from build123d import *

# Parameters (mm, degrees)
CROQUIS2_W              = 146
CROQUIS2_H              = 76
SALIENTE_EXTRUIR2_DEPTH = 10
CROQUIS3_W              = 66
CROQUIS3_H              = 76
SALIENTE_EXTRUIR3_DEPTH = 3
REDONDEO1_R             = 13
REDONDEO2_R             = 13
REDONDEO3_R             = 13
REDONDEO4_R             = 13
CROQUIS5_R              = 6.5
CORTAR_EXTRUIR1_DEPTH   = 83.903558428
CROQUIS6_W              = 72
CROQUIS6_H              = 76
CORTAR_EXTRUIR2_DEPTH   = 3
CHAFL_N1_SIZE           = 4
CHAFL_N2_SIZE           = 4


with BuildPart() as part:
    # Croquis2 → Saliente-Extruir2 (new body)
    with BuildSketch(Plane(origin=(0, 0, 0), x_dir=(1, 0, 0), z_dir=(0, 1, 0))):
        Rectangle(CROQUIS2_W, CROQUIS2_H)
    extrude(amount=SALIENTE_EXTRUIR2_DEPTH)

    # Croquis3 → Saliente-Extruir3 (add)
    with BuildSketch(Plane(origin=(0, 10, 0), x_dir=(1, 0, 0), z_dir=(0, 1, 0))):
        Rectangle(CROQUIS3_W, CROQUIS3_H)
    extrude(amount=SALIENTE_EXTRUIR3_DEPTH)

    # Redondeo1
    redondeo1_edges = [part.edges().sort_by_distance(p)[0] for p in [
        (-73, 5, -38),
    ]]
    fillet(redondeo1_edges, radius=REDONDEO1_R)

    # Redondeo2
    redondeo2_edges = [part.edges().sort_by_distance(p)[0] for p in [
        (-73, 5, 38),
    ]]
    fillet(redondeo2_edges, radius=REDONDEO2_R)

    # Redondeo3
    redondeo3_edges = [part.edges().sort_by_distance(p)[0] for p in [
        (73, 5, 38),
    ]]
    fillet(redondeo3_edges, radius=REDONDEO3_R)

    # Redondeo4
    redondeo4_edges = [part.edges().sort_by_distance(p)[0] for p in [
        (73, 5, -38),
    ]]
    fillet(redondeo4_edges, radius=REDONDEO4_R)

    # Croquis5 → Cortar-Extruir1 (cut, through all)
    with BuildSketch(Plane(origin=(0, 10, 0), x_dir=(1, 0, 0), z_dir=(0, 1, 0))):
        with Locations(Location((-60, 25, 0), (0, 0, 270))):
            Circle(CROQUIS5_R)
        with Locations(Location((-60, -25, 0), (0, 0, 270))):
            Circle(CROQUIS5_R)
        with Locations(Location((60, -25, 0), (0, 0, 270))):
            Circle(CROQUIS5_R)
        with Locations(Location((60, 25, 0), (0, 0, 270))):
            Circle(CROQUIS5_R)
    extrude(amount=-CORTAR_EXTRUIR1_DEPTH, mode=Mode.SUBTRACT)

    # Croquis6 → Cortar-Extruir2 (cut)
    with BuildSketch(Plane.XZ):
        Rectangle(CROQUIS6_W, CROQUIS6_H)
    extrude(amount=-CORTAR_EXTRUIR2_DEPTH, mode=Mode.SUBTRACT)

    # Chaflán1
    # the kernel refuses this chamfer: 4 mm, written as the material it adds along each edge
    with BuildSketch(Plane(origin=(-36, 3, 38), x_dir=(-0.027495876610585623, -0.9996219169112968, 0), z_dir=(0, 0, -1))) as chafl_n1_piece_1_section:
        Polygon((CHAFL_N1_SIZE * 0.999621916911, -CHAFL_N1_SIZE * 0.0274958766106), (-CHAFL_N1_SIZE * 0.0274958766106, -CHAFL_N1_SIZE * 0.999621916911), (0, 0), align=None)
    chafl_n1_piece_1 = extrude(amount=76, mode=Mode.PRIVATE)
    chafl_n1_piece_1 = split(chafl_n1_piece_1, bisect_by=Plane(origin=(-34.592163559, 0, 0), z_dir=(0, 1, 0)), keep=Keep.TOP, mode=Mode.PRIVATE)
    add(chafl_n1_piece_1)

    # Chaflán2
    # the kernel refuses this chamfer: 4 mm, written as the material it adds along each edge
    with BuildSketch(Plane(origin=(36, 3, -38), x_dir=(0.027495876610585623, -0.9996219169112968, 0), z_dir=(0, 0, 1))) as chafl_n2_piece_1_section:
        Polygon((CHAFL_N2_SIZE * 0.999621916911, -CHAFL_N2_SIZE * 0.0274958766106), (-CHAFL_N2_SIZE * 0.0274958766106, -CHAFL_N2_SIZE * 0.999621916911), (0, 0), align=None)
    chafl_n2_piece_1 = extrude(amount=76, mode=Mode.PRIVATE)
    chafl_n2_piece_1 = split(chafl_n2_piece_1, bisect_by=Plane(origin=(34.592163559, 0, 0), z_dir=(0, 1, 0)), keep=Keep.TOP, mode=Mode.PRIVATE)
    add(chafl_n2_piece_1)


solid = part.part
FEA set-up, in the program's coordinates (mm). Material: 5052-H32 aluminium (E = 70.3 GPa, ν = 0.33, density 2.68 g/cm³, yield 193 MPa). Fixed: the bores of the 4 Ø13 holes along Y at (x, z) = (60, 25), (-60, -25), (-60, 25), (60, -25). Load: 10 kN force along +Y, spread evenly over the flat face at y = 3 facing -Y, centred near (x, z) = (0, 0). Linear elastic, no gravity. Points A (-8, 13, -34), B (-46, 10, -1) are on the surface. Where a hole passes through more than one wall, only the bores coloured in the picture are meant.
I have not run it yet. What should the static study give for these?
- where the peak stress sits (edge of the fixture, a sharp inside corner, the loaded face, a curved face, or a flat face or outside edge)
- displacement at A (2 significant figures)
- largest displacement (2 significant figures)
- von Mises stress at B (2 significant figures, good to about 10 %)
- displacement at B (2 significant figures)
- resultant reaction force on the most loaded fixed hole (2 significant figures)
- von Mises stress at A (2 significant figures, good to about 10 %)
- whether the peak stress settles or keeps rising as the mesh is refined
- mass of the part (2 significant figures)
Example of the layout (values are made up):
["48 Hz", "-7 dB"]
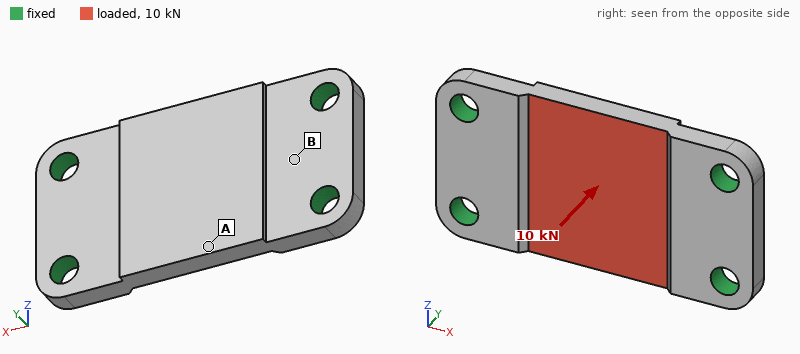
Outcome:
["edge of the fixture", "0.12 mm", "0.13 mm", "25 MPa", "0.025 mm", "4.5 kN", "63 MPa", "keeps rising", "280 g"]
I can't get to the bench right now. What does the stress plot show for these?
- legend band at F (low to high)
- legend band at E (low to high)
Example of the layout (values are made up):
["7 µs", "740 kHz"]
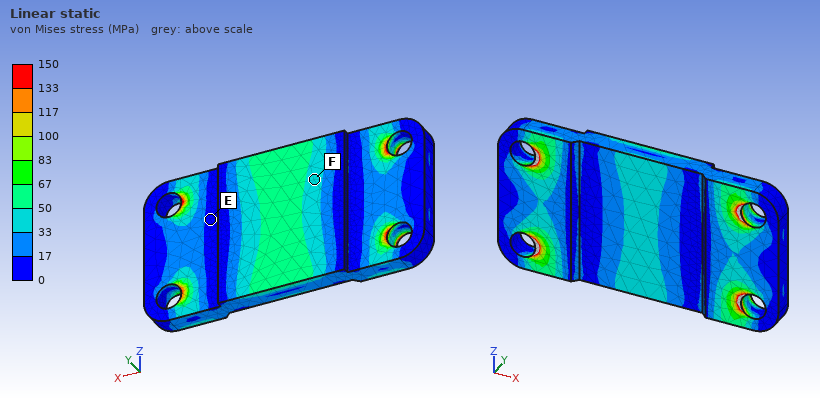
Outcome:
["33 to 50 MPa", "0 to 17 MPa"]
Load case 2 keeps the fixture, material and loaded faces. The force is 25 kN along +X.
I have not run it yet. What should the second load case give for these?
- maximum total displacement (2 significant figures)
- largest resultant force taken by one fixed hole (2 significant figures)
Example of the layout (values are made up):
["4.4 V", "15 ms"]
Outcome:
["18 µm", "6.4 kN"]
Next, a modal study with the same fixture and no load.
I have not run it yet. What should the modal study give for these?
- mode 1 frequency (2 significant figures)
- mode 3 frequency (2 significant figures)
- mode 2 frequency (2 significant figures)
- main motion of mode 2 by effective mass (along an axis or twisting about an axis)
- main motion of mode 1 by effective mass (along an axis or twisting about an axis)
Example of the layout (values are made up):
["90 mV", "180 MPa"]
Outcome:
["4200 Hz", "9600 Hz", "5500 Hz", "twisting about X", "along Y"]
